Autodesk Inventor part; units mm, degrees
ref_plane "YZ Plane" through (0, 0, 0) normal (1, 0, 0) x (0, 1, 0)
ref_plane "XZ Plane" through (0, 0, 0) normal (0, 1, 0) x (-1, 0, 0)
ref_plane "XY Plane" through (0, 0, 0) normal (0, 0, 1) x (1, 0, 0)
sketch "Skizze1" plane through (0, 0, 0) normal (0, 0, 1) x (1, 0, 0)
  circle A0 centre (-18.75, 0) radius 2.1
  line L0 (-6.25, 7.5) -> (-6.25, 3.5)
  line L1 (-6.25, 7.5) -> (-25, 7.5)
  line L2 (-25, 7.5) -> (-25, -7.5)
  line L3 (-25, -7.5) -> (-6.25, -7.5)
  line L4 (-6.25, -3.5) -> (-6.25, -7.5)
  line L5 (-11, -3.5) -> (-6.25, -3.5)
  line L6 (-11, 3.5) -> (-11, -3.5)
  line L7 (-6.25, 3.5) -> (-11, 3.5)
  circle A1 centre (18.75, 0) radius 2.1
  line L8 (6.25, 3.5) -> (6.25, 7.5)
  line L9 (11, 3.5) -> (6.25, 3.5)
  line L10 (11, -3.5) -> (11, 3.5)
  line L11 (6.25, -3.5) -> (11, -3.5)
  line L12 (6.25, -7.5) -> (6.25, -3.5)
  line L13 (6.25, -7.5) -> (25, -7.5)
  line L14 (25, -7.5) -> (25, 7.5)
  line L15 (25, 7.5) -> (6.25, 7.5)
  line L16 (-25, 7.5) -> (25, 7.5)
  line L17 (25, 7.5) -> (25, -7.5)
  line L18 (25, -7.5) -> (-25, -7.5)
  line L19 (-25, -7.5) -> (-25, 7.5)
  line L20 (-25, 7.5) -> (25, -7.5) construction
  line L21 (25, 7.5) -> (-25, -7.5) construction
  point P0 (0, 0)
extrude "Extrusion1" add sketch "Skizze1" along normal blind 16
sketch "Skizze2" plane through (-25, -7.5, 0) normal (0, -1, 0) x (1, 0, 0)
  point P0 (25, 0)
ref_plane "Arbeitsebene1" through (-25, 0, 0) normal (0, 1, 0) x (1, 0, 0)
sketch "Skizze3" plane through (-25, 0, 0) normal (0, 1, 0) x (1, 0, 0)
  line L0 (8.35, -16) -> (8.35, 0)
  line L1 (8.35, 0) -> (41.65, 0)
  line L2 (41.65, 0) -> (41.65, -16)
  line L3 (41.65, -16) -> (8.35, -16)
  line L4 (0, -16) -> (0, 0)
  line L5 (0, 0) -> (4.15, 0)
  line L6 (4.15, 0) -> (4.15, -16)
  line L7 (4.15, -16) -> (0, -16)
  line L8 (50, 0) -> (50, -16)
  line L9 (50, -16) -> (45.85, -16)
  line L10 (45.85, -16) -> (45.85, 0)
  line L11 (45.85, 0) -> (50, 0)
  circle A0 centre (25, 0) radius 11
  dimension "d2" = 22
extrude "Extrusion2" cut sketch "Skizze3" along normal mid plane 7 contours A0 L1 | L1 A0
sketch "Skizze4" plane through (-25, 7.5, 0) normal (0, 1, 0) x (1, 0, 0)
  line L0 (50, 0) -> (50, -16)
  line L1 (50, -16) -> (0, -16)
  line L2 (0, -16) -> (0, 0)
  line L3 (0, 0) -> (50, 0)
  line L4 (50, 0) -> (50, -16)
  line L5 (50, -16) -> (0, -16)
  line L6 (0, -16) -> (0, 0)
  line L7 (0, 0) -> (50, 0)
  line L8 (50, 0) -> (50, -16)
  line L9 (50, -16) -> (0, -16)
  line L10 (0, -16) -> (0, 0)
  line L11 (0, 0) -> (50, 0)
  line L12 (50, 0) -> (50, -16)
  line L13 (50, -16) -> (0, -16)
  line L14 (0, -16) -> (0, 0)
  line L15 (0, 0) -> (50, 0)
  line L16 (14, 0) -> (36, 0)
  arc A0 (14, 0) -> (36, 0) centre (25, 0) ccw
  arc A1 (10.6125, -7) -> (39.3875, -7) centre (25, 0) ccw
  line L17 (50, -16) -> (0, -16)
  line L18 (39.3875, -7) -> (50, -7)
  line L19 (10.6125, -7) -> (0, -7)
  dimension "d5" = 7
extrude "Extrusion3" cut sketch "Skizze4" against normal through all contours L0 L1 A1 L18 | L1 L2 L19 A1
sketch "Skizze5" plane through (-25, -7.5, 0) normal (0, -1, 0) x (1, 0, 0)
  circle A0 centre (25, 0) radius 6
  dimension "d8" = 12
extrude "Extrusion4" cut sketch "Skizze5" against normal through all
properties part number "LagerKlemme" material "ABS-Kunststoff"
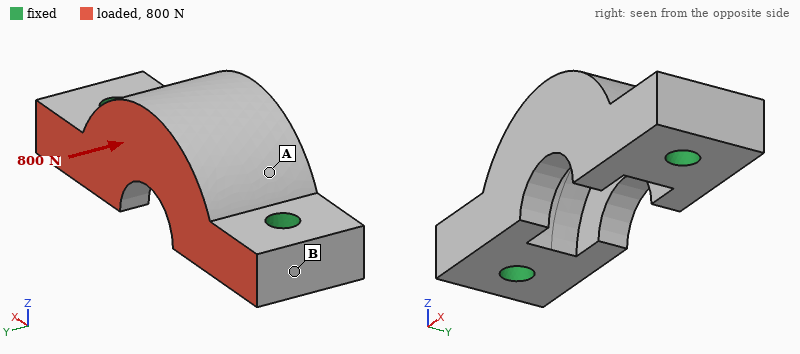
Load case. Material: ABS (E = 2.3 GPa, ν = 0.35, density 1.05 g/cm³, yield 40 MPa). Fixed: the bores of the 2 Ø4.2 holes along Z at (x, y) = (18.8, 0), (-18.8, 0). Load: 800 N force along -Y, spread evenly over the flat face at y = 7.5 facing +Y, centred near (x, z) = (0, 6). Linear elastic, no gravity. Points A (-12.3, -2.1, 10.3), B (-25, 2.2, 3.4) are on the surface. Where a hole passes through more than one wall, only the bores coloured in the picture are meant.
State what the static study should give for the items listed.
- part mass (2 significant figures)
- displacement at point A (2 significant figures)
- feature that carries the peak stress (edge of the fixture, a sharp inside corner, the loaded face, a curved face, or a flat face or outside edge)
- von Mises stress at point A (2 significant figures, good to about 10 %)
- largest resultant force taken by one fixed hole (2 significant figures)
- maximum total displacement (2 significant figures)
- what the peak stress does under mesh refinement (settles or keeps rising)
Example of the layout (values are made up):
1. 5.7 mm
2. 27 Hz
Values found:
1. 6.4 g
2. 0.099 mm
3. edge of the fixture
4. 7.6 MPa
5. 400 N
6. 0.20 mm
7. keeps rising
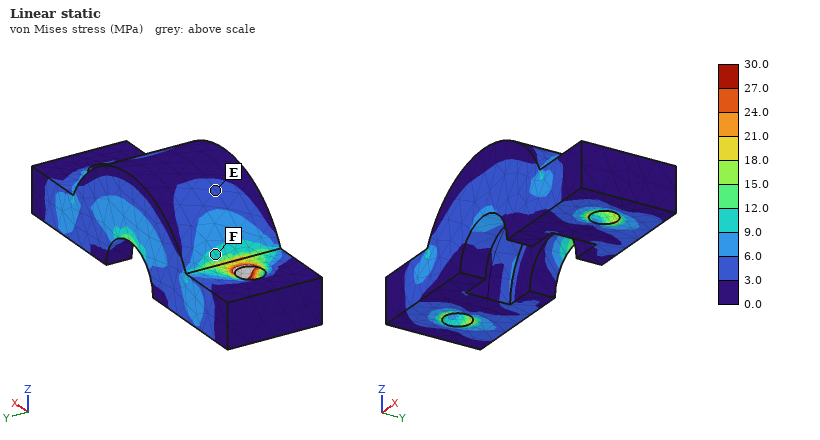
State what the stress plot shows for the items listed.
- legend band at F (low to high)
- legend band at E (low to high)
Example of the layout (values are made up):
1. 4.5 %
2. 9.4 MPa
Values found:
1. 9.0 to 12.0 MPa
2. 3.0 to 6.0 MPa
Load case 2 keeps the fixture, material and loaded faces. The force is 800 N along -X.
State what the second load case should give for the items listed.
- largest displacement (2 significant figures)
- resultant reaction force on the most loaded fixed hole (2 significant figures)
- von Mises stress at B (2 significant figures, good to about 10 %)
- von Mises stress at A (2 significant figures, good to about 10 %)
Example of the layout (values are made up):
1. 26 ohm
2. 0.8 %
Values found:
1. 85 µm
2. 420 N
3. 4.9 MPa
4. 2.3 MPa
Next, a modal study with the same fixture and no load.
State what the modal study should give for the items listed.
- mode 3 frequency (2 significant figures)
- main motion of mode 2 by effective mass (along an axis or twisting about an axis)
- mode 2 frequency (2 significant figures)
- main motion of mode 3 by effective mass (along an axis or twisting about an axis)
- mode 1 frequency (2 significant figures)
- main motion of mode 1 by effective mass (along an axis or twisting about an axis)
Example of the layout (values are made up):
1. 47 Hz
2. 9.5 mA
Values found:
1. 10 kHz
2. along Z
3. 7900 Hz
4. along Y
5. 4600 Hz
6. along Y
